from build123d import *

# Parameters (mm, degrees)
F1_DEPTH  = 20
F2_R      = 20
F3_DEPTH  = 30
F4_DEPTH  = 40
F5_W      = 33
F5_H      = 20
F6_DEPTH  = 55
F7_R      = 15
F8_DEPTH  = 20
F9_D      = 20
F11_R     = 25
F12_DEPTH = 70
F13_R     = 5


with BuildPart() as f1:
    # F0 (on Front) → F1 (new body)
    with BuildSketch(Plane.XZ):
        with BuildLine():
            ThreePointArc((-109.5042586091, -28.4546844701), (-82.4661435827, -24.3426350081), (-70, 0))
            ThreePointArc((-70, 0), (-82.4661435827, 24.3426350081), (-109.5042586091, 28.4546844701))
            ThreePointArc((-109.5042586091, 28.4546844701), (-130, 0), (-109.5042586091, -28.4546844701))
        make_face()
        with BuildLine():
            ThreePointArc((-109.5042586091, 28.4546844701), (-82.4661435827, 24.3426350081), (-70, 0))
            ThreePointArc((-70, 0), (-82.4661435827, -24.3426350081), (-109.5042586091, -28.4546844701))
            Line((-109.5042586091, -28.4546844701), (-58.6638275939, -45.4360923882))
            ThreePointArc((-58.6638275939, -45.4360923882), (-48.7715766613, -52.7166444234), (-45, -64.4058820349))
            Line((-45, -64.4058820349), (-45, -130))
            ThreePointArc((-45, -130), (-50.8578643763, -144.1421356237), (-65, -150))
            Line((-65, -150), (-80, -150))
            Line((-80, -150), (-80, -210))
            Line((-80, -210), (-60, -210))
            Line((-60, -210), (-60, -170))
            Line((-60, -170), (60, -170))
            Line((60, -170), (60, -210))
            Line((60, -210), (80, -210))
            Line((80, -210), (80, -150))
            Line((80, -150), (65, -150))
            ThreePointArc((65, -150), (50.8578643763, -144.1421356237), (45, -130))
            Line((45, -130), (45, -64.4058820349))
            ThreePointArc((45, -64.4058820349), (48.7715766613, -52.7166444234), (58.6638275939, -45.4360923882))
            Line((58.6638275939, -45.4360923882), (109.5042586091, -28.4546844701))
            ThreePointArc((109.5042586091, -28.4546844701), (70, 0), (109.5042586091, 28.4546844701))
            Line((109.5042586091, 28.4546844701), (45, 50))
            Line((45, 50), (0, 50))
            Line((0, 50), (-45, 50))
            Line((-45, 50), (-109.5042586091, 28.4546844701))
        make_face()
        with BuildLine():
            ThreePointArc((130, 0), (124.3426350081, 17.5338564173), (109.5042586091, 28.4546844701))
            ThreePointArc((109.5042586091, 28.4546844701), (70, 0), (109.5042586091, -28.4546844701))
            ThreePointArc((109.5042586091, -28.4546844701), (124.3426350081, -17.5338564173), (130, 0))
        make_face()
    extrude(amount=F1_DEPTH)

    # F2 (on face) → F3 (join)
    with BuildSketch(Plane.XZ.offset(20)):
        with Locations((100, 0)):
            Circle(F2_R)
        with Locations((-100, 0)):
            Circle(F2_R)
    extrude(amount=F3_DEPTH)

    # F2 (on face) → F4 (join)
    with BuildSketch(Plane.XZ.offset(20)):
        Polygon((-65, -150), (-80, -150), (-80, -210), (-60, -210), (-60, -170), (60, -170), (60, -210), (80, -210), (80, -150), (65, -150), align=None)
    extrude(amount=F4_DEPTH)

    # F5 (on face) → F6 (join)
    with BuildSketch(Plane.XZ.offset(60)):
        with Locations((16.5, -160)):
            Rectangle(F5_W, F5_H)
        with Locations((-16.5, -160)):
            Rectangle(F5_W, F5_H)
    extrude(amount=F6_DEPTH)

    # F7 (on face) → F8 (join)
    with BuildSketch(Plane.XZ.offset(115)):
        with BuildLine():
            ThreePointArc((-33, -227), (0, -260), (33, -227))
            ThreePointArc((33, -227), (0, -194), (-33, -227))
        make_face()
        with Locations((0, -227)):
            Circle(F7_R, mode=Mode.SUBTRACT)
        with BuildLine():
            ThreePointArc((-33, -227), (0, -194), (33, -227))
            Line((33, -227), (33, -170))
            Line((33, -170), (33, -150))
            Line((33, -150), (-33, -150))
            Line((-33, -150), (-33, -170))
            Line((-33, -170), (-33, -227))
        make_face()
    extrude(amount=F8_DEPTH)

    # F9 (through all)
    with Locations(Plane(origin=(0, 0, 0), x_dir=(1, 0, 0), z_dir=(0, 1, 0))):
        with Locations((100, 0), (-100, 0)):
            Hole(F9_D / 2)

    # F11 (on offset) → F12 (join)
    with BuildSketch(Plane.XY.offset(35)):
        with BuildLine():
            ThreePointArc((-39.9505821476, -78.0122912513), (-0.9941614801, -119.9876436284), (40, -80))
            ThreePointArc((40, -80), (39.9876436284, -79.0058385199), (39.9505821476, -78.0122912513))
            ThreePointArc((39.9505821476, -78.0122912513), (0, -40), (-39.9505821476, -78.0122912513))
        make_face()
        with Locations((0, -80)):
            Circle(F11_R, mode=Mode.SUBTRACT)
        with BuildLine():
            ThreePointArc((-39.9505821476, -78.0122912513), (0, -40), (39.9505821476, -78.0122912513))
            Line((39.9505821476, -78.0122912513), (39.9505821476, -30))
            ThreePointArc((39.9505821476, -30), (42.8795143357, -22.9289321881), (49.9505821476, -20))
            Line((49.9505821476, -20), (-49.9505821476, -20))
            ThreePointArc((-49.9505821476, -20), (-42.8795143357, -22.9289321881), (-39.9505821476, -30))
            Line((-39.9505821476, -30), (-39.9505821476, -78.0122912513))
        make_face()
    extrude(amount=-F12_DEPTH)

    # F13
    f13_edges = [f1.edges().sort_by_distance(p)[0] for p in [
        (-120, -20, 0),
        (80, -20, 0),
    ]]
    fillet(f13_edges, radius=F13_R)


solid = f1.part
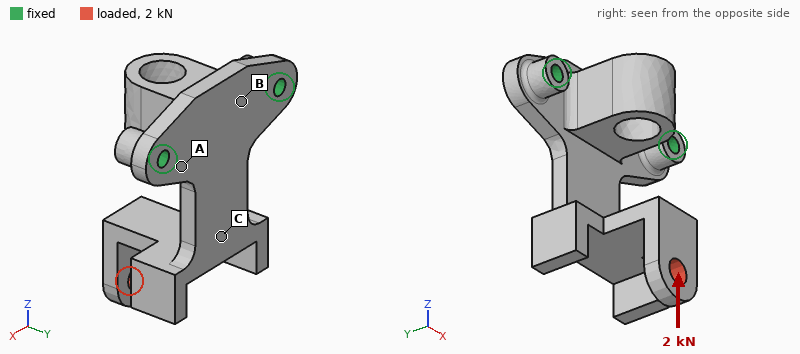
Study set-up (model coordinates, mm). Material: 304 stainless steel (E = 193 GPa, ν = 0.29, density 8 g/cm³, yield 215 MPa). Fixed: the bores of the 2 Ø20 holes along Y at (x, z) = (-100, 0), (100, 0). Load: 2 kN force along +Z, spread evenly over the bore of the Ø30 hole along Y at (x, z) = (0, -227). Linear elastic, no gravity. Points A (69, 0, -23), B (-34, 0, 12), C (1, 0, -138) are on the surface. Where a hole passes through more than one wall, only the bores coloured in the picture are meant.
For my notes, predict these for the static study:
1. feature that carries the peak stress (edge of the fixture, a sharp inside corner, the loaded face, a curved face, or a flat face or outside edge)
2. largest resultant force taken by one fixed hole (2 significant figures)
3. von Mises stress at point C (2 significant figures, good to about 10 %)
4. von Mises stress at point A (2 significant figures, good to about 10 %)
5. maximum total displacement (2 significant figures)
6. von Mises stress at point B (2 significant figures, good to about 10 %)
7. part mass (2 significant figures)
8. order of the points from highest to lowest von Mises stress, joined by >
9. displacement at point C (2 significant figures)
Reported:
a curved face
1.0 kN
31 MPa
15 MPa
0.74 mm
6.2 MPa
12 kg
C > A > B
0.16 mm
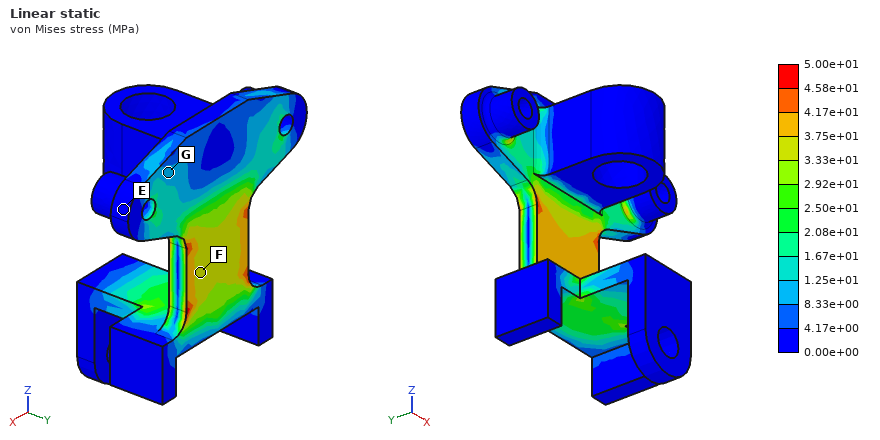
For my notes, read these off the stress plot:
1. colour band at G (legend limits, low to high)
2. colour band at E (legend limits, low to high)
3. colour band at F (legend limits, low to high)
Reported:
8.33e+00 to 1.25e+01 MPa
0.00e+00 to 4.17e+00 MPa
3.33e+01 to 3.75e+01 MPa
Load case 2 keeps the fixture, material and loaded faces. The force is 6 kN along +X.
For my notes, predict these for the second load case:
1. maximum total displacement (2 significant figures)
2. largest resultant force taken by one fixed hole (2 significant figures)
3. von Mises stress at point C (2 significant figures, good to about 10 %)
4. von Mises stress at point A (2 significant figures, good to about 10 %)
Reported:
0.88 mm
9.4 kN
53 MPa
32 MPa
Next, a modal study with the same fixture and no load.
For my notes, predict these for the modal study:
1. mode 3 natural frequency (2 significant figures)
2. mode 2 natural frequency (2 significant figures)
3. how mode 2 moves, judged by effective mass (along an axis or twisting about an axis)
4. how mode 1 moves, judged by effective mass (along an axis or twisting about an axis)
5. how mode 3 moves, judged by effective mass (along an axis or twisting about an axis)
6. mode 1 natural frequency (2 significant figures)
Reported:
590 Hz
370 Hz
along X
along Y
along Y
180 Hz
